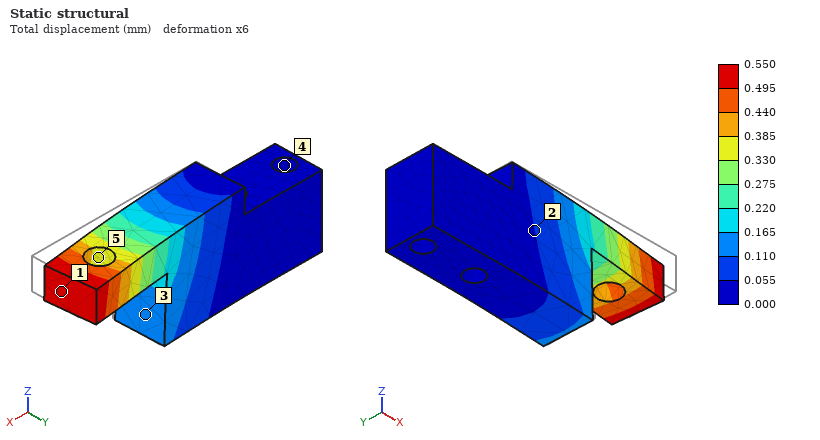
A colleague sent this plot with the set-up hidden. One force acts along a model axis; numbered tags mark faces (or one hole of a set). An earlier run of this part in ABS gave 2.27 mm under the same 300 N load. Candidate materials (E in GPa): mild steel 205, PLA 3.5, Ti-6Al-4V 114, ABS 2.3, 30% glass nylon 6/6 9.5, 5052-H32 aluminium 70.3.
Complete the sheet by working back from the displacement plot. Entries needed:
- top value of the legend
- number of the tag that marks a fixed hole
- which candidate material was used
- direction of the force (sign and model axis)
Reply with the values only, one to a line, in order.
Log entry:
0.550 mm
4
30% glass nylon 6/6
+Y
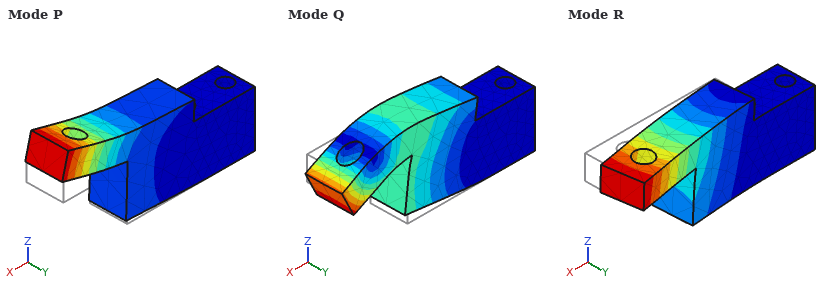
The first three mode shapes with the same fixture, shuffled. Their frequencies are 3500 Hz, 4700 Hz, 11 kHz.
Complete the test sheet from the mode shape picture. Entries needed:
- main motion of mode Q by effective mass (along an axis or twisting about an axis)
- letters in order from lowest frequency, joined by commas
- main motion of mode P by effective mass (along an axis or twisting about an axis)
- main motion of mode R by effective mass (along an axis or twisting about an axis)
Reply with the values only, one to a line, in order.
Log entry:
along Z
R, P, Q
along Z
along Y
